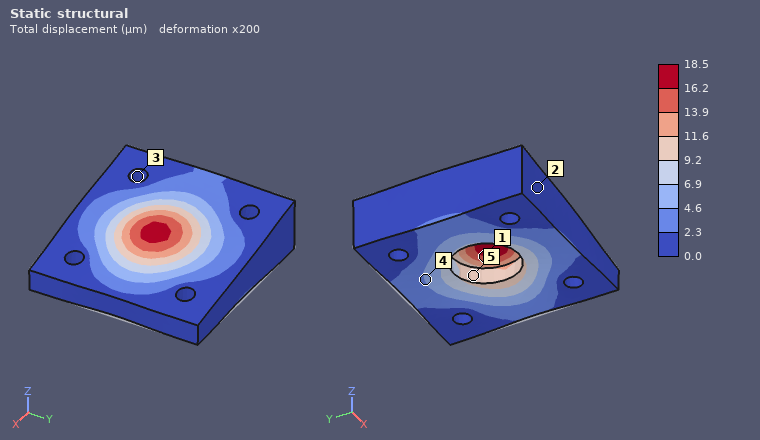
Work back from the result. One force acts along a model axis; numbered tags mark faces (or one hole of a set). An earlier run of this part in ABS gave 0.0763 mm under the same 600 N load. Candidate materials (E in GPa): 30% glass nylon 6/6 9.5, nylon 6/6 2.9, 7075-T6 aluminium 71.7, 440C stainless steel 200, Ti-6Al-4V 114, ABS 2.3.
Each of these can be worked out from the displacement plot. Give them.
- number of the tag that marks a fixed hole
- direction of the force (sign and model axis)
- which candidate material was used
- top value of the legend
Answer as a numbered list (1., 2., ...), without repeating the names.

1. 3
2. +Z
3. 30% glass nylon 6/6
4. 18.5 µm
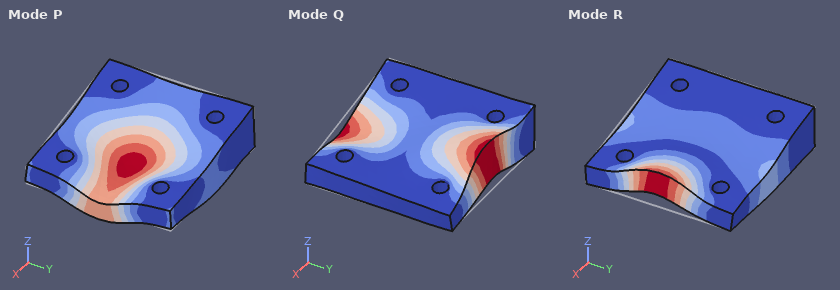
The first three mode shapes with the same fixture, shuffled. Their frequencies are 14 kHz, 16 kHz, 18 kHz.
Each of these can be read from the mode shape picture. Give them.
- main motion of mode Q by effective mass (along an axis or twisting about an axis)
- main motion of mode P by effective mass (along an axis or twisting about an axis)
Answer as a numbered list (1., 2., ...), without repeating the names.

1. twisting about X
2. along Z
